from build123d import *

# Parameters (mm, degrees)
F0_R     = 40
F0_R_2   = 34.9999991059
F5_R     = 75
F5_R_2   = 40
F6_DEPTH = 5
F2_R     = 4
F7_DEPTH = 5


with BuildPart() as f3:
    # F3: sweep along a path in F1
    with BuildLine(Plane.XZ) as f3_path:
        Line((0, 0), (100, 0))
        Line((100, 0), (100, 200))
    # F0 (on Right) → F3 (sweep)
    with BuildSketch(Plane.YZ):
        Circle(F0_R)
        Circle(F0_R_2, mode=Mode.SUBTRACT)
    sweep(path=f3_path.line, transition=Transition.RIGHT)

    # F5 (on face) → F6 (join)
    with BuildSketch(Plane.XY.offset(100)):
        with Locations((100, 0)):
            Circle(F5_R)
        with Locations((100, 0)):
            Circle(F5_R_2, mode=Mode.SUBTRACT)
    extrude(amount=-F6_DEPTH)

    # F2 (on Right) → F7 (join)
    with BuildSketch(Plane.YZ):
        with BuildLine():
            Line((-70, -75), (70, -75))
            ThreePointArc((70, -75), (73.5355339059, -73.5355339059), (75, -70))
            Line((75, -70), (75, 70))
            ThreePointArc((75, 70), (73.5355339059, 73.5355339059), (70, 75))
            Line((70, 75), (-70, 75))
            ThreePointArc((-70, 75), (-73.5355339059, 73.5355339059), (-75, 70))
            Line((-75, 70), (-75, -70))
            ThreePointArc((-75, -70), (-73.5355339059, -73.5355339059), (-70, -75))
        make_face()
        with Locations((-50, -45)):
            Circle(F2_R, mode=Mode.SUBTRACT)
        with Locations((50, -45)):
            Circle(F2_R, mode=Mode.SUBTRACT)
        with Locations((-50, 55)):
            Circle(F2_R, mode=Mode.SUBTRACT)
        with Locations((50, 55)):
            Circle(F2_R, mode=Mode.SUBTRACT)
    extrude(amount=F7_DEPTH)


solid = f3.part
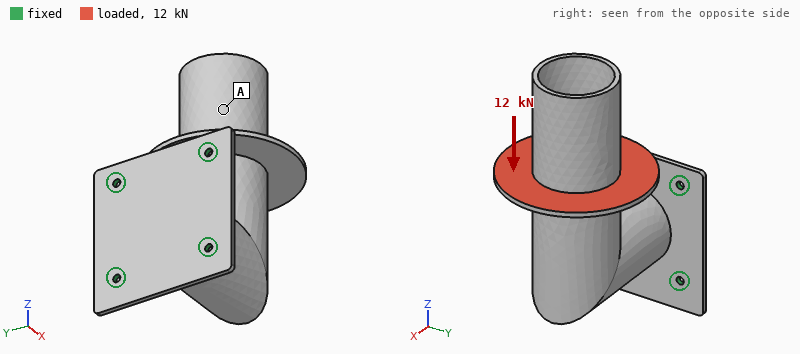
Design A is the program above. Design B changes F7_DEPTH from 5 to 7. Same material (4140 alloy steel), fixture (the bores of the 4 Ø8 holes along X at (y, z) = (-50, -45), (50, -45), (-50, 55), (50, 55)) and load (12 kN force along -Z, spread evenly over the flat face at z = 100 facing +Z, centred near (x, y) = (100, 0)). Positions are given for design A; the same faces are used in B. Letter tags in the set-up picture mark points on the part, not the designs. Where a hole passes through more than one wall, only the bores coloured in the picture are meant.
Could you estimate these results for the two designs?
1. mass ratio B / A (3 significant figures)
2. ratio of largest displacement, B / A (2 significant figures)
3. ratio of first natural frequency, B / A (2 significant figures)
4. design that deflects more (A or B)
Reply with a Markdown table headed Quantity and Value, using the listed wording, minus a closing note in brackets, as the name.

| Quantity | Value |
|---|---|
| mass ratio B / A | 1.08 |
| ratio of largest displacement, B / A | 0.48 |
| ratio of first natural frequency, B / A | 1.4 |
| design that deflects more | A |
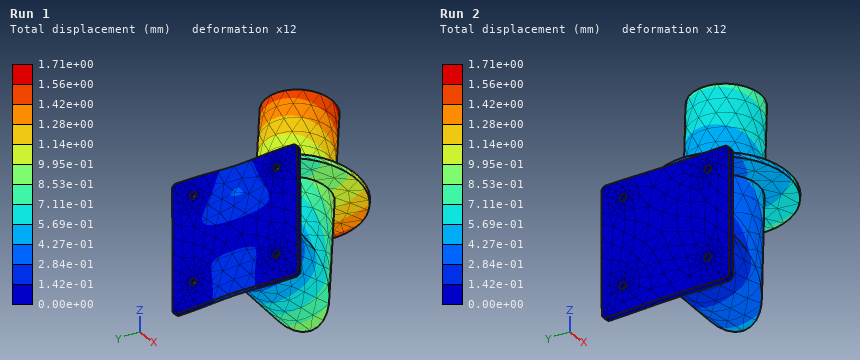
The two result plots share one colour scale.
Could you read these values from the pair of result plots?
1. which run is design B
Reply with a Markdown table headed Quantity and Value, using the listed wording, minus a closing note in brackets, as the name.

| Quantity | Value |
|---|---|
| which run is design B | Run 2 |
